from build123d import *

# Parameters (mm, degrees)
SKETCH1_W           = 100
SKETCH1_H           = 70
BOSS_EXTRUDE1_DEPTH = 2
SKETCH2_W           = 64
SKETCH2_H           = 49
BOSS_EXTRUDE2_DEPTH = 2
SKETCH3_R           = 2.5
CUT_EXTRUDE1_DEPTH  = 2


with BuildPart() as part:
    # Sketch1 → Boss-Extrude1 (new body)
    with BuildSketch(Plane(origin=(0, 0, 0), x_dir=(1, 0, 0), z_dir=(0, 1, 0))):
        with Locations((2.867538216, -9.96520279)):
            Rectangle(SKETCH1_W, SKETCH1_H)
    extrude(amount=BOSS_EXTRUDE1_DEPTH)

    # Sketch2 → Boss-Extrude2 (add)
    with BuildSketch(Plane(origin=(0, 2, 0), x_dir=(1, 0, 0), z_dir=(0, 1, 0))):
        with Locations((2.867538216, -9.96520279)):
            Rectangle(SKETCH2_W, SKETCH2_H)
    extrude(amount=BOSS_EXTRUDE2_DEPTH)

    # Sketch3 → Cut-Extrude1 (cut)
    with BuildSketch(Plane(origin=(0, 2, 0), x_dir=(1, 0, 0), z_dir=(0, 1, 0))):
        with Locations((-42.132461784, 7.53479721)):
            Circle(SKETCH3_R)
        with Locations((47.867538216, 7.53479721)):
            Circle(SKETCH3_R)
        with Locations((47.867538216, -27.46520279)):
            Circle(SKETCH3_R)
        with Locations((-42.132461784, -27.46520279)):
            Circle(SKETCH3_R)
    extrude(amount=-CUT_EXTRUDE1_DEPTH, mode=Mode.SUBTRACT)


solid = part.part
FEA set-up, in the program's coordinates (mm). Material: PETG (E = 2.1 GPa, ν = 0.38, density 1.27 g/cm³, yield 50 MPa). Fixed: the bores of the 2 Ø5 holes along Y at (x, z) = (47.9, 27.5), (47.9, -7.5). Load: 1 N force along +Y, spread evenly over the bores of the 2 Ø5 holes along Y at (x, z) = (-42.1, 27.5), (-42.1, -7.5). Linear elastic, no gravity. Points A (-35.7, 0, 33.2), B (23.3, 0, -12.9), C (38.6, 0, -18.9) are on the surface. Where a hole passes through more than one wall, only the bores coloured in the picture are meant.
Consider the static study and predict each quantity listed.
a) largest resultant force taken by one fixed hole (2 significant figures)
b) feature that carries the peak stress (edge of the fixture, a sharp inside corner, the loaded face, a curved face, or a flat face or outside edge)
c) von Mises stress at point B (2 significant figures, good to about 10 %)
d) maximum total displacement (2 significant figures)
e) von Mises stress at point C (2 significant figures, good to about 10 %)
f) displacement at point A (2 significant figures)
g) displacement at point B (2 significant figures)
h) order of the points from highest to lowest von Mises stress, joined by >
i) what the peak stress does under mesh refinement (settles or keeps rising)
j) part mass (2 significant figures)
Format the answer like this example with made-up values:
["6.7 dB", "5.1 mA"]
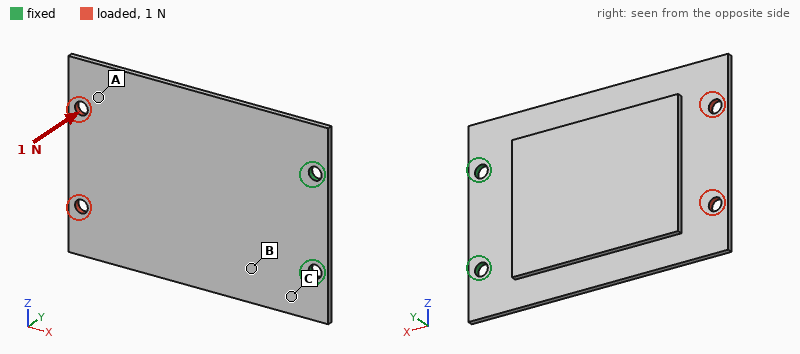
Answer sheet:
["1.0 N", "edge of the fixture", "0.45 MPa", "1.3 mm", "1.4 MPa", "1.1 mm", "0.22 mm", "C > B > A", "keeps rising", "26 g"]
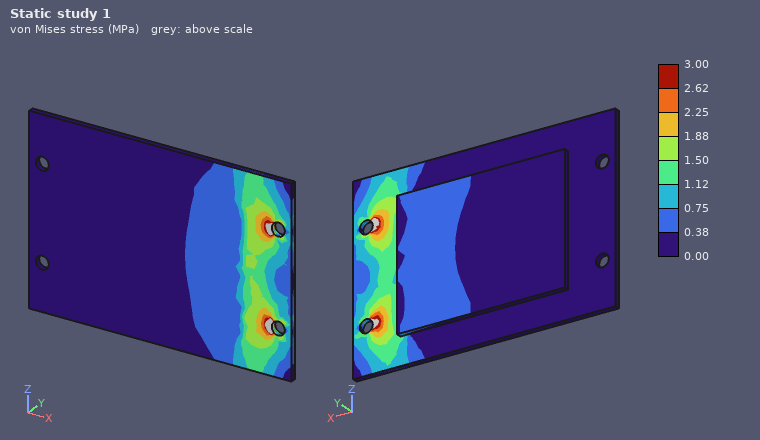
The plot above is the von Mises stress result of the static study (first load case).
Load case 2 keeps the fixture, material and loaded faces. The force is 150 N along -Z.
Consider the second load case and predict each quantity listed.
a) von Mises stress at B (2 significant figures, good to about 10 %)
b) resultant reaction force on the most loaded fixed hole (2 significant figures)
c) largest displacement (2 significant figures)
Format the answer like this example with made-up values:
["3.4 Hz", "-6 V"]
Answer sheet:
["4.6 MPa", "360 N", "1.2 mm"]
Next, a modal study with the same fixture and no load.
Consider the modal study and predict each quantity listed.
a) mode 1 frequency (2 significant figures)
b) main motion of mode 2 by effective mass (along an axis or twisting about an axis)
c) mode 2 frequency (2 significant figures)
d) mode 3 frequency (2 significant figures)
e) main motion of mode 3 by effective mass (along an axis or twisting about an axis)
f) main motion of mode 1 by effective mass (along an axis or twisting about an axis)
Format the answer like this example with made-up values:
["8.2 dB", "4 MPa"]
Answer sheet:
["53 Hz", "twisting about X", "240 Hz", "480 Hz", "along Y", "along Y"]
